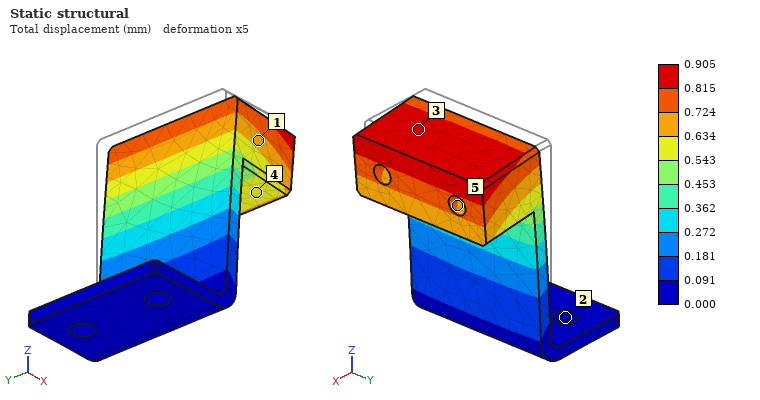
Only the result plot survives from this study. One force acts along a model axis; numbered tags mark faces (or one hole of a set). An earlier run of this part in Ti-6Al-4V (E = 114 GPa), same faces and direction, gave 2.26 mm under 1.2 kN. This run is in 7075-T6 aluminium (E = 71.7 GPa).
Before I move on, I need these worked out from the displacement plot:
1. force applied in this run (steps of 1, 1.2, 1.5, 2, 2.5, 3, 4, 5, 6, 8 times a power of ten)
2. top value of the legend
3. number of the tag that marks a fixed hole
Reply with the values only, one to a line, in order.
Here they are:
300 N
0.905 mm
2
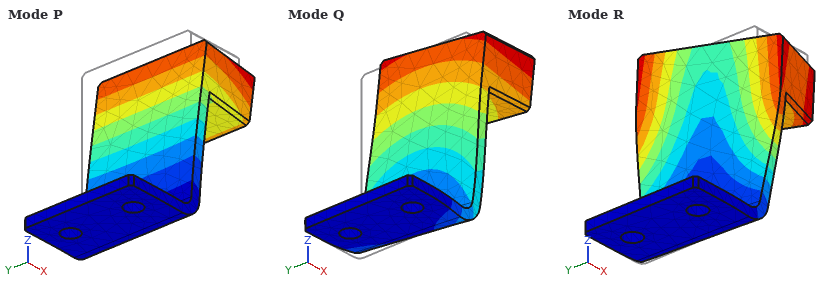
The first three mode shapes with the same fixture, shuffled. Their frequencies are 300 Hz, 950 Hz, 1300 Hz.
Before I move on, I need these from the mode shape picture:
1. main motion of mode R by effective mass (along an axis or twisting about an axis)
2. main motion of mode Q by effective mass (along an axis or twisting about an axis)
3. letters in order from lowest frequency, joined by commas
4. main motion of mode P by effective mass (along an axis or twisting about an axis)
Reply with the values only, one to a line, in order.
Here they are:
twisting about Z
along Y
P, Q, R
along X
